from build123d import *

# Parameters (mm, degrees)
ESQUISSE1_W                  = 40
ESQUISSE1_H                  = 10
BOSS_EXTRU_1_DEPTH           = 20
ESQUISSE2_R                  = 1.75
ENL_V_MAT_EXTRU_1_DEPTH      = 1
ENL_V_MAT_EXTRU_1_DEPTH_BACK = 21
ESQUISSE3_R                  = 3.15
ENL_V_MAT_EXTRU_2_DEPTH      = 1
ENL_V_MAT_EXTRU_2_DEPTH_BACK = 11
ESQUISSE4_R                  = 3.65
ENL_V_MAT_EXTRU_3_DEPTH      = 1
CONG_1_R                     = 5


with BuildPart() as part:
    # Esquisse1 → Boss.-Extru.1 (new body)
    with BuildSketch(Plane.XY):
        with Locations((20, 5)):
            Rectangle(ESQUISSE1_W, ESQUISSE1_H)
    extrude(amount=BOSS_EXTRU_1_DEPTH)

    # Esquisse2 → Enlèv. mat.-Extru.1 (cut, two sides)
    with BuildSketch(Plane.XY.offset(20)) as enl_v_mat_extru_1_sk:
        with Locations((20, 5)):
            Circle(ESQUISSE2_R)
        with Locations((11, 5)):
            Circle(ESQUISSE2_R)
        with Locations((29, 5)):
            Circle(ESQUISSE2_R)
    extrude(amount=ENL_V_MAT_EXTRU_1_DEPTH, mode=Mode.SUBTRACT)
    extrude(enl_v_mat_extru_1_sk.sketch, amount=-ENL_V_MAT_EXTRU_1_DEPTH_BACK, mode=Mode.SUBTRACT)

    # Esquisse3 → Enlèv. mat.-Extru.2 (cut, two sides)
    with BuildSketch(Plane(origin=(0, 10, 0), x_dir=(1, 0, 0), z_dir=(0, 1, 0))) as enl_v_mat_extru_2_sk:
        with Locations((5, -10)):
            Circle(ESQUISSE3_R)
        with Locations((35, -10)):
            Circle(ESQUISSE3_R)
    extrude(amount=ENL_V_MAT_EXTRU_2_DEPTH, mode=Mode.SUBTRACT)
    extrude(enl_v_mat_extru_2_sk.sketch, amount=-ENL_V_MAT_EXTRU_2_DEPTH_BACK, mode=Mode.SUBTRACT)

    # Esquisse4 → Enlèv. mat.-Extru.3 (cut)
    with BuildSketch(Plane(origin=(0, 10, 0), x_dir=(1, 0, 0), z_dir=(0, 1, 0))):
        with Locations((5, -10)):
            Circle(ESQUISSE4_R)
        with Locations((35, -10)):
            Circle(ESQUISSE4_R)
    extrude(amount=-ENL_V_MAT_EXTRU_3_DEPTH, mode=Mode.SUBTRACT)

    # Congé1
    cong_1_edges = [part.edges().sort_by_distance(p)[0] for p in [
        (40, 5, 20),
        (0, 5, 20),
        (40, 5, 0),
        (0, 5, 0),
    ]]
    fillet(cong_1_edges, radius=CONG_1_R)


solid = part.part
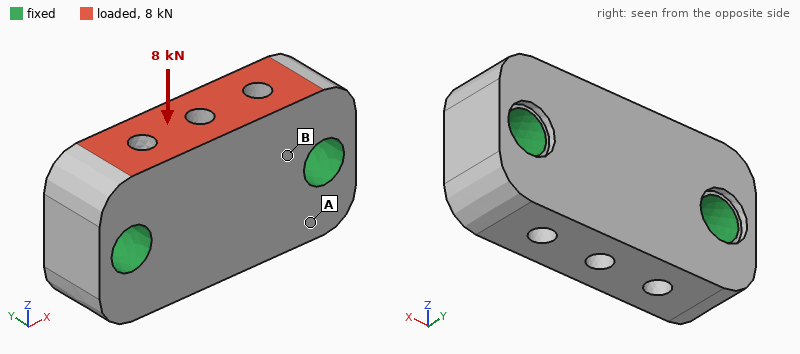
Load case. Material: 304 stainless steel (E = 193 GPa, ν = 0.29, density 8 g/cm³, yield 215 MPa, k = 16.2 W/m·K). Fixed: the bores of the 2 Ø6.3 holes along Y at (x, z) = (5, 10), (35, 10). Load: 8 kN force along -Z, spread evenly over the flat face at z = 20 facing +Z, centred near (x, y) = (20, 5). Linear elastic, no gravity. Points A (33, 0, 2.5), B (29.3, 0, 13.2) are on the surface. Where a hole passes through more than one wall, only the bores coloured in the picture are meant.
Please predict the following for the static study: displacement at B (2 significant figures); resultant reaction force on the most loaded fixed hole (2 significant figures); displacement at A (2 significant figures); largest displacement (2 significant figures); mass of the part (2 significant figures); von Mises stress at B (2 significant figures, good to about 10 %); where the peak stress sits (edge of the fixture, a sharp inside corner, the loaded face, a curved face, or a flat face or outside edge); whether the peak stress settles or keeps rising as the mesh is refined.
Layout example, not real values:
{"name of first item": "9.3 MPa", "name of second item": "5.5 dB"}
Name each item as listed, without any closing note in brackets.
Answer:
{"displacement at B": "1.7 µm", "resultant reaction force on the most loaded fixed hole": "4.1 kN", "displacement at A": "0.84 µm", "largest displacement": "4.6 µm", "mass of the part": "53 g", "von Mises stress at B": "45 MPa", "where the peak stress sits": "edge of the fixture", "whether the peak stress settles or keeps rising as the mesh is refined": "keeps rising"}
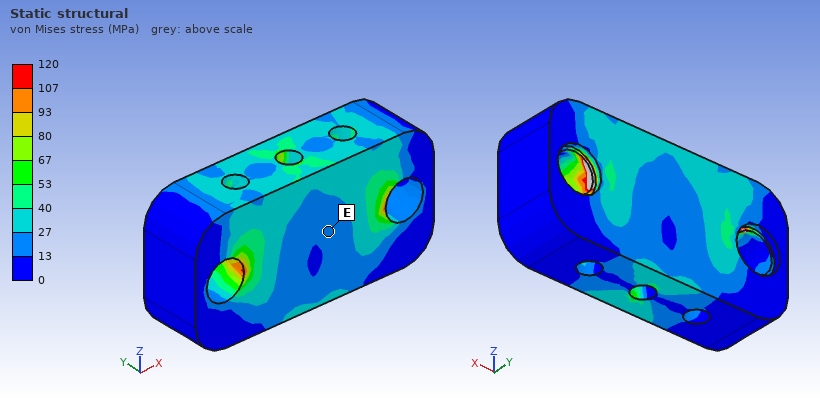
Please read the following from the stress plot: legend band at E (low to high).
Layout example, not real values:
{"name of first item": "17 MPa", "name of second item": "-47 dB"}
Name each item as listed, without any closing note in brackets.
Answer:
{"legend band at E": "13 to 27 MPa"}
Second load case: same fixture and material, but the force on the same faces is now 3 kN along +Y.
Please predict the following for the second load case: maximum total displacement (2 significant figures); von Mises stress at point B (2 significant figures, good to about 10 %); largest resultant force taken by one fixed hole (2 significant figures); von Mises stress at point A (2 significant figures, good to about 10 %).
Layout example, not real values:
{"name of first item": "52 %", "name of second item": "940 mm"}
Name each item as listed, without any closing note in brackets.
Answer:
{"maximum total displacement": "8.0 µm", "von Mises stress at point B": "46 MPa", "largest resultant force taken by one fixed hole": "1.5 kN", "von Mises stress at point A": "10 MPa"}
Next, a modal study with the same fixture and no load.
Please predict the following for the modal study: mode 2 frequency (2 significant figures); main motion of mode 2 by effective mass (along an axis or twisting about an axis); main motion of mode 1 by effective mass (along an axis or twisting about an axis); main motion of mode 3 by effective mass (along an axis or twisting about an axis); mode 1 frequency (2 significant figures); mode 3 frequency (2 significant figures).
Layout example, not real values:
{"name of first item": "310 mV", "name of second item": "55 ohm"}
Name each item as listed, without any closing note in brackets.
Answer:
{"mode 2 frequency": "36 kHz", "main motion of mode 2 by effective mass": "twisting about X", "main motion of mode 1 by effective mass": "along Y", "main motion of mode 3 by effective mass": "along Z", "mode 1 frequency": "32 kHz", "mode 3 frequency": "40 kHz"}
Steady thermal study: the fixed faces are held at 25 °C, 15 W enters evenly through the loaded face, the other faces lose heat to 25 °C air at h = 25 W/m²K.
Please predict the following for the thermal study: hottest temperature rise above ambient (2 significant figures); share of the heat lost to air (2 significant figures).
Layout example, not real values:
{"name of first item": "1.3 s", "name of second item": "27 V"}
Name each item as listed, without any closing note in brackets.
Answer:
{"hottest temperature rise above ambient": "41 K", "share of the heat lost to air": "5.3 %"}
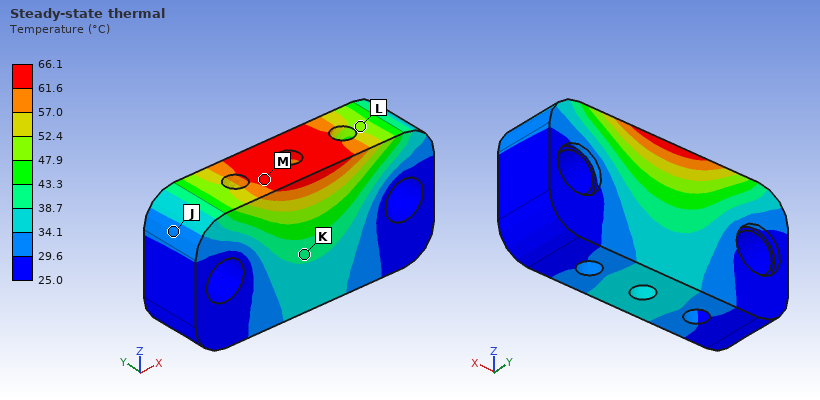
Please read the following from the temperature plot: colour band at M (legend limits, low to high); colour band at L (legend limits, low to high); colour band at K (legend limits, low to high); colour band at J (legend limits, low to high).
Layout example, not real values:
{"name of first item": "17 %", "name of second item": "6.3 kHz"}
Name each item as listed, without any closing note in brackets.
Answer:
{"colour band at M": "61.6 to 66.1 °C", "colour band at L": "47.9 to 52.4 °C", "colour band at K": "38.7 to 43.3 °C", "colour band at J": "29.6 to 34.1 °C"}
